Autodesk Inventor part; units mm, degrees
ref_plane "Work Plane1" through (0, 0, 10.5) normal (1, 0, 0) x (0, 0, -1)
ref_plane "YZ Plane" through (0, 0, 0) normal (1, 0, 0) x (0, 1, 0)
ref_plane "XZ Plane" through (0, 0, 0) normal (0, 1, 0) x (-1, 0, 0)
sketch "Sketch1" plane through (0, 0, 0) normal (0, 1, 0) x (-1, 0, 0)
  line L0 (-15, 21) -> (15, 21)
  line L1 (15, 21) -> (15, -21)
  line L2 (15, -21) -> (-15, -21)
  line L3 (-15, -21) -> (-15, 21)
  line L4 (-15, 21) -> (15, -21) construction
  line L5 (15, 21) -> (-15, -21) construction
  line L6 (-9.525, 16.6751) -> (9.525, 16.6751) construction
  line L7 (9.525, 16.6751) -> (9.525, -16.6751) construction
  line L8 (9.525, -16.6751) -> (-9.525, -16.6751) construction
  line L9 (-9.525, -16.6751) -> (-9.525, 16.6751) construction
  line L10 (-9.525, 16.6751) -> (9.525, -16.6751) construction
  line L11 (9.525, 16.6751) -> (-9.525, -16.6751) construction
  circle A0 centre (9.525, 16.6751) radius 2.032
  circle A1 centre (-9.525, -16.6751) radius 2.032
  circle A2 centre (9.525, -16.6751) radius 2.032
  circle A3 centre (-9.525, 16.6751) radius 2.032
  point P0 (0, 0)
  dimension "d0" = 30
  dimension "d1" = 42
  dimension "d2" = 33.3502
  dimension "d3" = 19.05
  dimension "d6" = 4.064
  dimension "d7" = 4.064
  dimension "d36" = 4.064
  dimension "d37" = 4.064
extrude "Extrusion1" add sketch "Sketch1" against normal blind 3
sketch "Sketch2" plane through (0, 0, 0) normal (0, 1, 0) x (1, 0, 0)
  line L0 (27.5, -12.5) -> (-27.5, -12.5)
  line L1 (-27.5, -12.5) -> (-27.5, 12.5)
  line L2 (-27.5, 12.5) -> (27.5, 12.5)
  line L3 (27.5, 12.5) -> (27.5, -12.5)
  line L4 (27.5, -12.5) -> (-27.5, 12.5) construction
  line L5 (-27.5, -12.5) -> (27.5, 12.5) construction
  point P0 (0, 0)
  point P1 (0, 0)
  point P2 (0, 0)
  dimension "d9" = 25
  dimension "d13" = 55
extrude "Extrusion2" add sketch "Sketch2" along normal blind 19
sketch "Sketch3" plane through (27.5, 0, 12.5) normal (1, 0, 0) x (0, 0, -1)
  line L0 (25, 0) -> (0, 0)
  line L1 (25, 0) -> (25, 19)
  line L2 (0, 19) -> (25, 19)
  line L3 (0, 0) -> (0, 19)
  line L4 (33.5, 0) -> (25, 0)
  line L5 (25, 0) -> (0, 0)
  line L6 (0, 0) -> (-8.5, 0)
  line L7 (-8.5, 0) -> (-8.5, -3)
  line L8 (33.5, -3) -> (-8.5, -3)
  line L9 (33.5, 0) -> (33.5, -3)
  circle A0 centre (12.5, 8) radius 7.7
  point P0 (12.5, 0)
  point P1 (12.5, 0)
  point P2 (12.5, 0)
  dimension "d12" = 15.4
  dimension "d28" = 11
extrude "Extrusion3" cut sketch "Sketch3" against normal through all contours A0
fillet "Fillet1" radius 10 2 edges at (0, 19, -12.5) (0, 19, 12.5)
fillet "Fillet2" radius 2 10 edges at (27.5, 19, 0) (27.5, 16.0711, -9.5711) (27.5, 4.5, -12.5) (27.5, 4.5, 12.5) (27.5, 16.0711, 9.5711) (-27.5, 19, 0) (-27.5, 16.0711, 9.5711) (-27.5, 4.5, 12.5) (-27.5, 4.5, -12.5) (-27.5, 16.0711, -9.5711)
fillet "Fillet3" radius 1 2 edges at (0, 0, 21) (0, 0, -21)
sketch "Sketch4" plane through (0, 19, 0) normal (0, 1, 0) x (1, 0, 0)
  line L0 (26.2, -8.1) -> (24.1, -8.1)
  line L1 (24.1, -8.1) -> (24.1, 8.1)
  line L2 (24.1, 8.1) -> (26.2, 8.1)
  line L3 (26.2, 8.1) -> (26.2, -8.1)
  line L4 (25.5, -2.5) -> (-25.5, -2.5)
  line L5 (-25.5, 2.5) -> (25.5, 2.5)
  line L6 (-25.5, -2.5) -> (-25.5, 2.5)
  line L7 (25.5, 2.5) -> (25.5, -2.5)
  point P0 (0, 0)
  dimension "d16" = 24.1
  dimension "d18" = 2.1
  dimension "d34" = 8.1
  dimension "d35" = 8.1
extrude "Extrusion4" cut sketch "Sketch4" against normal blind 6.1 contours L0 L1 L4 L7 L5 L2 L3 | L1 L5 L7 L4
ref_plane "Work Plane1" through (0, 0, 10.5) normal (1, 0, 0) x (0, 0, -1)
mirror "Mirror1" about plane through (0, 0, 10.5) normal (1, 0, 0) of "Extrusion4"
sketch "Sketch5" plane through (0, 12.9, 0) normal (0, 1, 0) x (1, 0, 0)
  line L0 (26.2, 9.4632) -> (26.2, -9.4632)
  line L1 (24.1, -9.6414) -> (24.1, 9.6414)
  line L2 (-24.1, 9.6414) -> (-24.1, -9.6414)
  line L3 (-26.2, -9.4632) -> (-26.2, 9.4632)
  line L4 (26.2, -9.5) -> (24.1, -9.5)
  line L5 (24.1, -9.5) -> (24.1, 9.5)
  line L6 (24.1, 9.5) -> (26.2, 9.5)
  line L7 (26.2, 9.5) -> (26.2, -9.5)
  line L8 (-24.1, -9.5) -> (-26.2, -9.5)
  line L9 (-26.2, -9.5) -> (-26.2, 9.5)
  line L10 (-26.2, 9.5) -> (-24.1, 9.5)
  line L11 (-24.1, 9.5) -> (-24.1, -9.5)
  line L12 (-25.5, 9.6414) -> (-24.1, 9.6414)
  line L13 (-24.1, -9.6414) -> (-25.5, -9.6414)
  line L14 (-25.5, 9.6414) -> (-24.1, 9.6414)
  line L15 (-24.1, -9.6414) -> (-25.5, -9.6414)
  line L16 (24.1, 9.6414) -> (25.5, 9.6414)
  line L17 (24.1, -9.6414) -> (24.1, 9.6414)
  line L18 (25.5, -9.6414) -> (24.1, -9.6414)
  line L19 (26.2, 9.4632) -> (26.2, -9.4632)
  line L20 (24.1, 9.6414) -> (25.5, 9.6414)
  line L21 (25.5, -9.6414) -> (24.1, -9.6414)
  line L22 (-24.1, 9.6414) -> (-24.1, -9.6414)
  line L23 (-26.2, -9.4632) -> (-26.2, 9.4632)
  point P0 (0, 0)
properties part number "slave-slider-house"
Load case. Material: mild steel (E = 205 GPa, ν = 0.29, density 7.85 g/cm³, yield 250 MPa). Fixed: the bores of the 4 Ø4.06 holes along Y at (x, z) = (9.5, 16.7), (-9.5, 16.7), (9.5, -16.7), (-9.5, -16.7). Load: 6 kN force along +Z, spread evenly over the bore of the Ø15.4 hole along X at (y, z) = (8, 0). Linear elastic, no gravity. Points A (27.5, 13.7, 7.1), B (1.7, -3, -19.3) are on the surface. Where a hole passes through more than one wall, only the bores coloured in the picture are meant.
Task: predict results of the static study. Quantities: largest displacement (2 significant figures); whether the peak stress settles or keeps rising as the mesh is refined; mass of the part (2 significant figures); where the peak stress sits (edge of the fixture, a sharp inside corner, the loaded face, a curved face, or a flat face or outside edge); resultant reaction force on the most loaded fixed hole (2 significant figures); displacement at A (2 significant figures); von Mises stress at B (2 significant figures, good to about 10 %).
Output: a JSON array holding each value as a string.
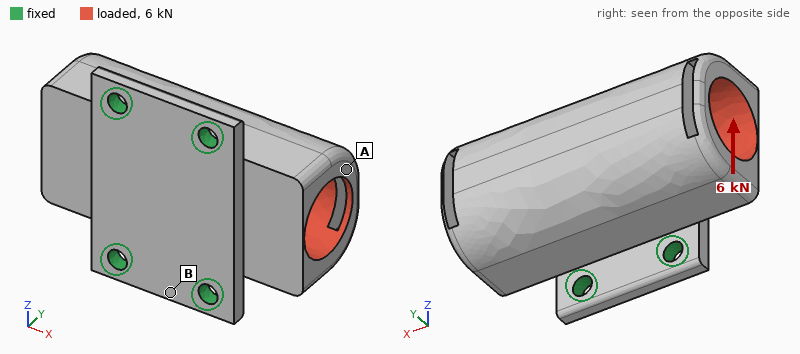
["13 µm", "keeps rising", "130 g", "edge of the fixture", "1.8 kN", "12 µm", "21 MPa"]
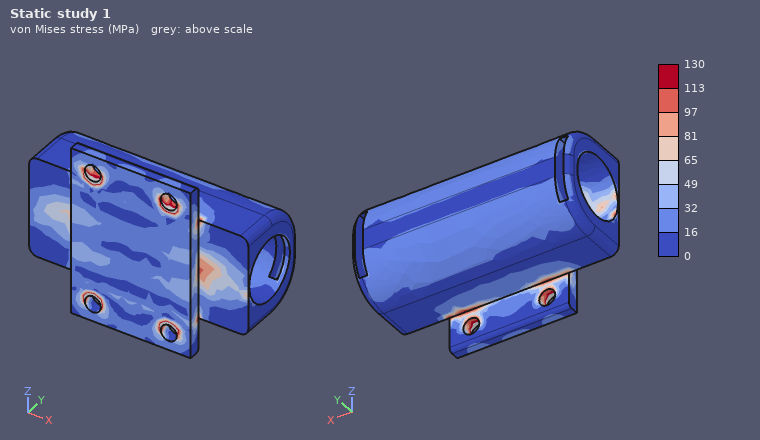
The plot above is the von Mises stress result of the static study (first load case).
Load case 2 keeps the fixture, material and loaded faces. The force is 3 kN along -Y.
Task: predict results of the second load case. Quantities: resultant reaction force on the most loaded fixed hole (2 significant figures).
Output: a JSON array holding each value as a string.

["810 N"]
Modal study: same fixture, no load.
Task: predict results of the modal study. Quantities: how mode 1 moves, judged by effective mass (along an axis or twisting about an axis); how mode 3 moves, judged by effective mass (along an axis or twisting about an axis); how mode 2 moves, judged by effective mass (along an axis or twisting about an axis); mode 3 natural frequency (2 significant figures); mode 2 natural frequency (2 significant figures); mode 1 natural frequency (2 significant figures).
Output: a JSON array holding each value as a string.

["along X", "along Y", "along Z", "13 kHz", "12 kHz", "7100 Hz"]
